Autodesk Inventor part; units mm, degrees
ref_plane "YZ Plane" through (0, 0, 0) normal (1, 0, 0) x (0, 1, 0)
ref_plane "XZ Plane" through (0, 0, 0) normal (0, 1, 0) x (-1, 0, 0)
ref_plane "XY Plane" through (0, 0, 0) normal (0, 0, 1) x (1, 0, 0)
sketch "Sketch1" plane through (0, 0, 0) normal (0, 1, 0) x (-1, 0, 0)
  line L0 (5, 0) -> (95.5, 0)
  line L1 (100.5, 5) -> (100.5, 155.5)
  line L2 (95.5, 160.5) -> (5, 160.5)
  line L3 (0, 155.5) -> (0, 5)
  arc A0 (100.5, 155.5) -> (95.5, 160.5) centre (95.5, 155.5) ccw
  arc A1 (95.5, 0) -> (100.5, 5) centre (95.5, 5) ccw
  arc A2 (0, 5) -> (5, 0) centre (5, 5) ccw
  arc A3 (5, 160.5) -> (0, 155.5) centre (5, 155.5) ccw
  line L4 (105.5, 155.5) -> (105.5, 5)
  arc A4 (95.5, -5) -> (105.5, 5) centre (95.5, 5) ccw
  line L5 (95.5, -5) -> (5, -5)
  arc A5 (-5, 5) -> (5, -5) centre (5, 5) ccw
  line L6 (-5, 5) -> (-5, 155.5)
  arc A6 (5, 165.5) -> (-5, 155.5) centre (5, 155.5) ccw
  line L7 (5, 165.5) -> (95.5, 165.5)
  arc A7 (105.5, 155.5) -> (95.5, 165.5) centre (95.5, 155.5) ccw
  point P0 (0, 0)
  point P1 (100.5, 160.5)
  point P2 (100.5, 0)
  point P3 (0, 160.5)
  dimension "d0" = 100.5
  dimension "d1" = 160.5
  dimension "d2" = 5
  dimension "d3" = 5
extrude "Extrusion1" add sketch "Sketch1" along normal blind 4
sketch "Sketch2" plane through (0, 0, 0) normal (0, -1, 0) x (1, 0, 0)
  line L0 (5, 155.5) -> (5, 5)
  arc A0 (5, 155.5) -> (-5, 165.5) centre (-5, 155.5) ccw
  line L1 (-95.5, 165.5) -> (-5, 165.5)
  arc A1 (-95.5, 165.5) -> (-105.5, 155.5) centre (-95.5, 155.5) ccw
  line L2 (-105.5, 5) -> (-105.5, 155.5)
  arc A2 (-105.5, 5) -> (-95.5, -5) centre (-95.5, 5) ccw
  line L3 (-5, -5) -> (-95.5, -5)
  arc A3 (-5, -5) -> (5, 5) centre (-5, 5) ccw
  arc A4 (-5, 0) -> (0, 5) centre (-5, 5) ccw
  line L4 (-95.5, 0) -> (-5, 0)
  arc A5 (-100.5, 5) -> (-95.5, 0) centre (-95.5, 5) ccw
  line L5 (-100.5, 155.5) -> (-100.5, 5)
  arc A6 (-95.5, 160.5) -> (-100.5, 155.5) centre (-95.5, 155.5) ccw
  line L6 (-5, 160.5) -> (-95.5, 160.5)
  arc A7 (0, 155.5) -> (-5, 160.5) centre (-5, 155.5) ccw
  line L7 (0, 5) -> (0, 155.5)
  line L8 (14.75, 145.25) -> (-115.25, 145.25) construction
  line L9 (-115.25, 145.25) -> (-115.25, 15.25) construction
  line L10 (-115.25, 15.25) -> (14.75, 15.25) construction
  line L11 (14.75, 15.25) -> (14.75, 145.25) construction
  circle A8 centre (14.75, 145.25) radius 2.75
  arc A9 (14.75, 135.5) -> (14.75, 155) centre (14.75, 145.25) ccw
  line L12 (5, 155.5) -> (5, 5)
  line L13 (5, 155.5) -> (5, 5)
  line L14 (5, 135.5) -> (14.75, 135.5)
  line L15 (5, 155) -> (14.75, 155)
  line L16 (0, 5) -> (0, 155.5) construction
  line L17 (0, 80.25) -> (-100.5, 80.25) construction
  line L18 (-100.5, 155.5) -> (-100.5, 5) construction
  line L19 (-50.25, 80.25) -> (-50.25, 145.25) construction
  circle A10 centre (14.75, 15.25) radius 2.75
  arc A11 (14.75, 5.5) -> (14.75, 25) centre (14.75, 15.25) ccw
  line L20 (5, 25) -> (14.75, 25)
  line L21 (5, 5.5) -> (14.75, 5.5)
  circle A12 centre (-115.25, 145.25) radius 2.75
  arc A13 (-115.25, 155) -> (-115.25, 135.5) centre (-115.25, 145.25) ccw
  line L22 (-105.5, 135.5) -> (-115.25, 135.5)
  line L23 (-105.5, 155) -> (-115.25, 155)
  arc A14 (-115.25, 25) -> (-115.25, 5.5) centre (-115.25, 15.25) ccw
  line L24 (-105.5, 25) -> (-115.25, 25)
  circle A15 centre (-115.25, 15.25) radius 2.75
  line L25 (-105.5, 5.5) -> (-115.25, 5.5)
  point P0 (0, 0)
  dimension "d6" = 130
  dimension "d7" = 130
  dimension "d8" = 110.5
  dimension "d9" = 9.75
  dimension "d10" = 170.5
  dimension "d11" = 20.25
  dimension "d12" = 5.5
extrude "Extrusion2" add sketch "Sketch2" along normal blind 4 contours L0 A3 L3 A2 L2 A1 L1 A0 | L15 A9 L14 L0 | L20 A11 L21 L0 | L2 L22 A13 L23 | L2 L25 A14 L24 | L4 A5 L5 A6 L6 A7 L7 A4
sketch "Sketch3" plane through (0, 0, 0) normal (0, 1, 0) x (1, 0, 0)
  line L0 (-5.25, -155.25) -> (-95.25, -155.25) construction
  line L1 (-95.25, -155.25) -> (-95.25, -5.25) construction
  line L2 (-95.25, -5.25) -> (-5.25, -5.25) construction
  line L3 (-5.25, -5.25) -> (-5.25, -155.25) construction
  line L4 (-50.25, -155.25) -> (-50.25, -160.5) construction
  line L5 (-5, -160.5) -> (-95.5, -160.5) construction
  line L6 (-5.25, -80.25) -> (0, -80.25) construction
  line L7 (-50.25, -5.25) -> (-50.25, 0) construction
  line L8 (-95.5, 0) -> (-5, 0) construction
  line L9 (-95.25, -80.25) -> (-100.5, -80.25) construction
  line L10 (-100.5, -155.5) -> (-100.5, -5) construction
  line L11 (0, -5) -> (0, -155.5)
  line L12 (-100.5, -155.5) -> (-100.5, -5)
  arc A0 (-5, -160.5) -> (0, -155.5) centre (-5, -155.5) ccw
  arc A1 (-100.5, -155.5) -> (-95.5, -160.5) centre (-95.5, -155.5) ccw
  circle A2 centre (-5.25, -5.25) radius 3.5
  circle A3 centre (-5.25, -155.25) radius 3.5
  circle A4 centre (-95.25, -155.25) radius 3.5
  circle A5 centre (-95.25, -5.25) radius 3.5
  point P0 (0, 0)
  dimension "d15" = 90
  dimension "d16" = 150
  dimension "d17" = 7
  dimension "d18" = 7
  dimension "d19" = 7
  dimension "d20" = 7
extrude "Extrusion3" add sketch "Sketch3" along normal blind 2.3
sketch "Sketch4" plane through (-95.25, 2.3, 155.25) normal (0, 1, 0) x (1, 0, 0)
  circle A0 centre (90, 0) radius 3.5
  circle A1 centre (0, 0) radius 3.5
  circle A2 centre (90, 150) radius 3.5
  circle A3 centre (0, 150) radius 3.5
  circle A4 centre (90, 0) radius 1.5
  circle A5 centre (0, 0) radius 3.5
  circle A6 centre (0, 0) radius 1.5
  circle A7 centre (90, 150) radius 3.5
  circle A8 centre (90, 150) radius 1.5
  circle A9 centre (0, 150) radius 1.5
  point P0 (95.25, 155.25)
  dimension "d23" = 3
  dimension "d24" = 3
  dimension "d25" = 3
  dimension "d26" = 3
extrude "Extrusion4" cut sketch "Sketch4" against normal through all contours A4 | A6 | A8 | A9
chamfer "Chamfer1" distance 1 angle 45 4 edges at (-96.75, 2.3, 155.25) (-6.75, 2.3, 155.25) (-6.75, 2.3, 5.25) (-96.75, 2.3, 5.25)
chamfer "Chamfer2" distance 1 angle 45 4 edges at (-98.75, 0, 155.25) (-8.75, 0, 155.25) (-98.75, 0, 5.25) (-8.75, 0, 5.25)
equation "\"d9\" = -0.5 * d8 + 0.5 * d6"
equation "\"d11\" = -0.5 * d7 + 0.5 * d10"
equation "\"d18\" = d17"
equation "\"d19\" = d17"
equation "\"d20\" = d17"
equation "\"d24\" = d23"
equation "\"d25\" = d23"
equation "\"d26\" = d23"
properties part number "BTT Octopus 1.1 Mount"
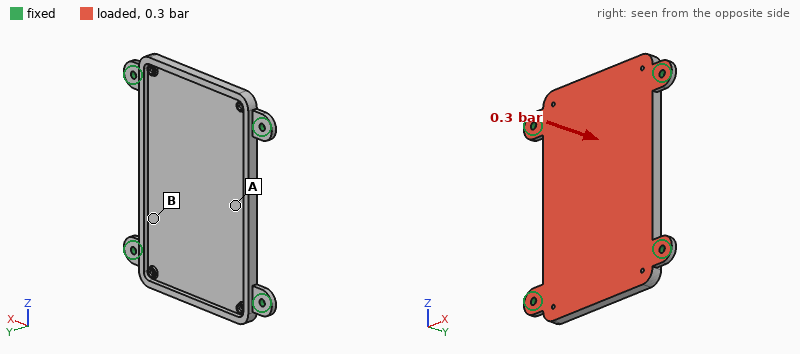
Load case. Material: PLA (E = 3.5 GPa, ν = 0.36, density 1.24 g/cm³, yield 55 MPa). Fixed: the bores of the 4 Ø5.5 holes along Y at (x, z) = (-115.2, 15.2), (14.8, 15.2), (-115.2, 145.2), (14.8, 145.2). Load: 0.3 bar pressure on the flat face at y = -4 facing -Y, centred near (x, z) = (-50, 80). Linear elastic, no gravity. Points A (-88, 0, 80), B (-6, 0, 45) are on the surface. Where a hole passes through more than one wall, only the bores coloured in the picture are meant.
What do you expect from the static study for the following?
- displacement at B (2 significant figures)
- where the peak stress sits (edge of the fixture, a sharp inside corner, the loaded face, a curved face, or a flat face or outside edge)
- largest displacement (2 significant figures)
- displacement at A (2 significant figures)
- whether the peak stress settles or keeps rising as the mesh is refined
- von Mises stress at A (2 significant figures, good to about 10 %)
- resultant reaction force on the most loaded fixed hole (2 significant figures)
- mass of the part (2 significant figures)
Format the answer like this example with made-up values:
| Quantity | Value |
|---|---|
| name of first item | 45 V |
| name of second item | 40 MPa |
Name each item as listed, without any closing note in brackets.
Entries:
| Quantity | Value |
|---|---|
| displacement at B | 1.3 mm |
| where the peak stress sits | edge of the fixture |
| largest displacement | 2.7 mm |
| displacement at A | 2.0 mm |
| whether the peak stress settles or keeps rising as the mesh is refined | keeps rising |
| von Mises stress at A | 6.0 MPa |
| resultant reaction force on the most loaded fixed hole | 160 N |
| mass of the part | 110 g |
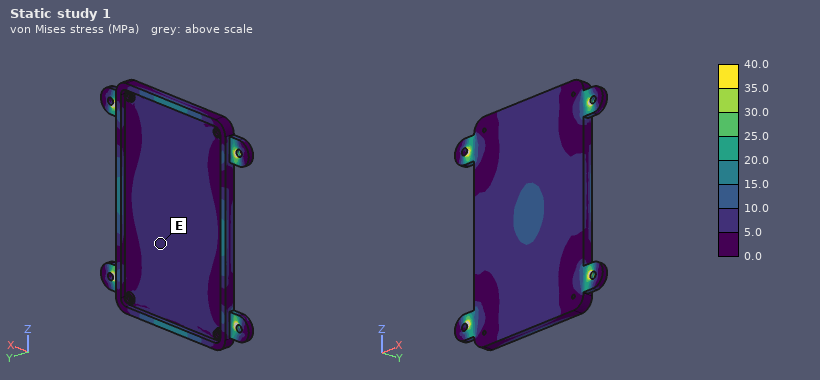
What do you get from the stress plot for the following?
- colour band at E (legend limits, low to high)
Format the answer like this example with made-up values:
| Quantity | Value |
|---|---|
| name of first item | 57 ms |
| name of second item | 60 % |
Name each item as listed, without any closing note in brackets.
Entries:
| Quantity | Value |
|---|---|
| colour band at E | 5.0 to 10.0 MPa |
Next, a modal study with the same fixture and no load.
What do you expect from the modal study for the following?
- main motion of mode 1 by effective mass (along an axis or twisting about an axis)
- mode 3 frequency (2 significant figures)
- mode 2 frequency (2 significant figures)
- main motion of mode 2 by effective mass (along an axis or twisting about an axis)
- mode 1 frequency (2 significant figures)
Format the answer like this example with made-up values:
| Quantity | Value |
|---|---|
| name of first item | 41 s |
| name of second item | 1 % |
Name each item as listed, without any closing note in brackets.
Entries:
| Quantity | Value |
|---|---|
| main motion of mode 1 by effective mass | along Y |
| mode 3 frequency | 500 Hz |
| mode 2 frequency | 450 Hz |
| main motion of mode 2 by effective mass | twisting about X |
| mode 1 frequency | 280 Hz |
